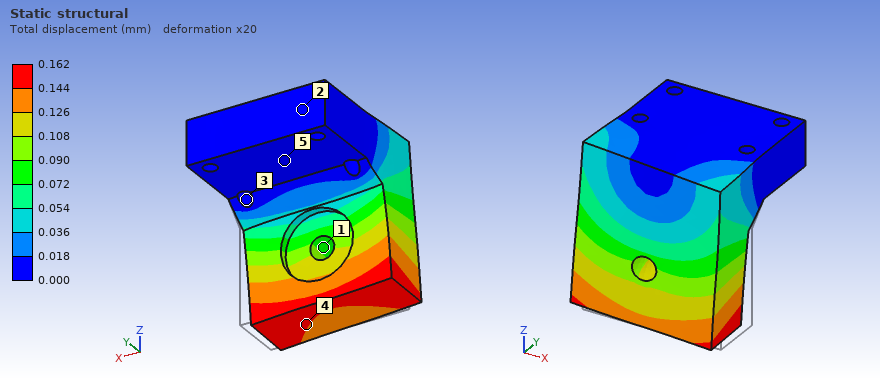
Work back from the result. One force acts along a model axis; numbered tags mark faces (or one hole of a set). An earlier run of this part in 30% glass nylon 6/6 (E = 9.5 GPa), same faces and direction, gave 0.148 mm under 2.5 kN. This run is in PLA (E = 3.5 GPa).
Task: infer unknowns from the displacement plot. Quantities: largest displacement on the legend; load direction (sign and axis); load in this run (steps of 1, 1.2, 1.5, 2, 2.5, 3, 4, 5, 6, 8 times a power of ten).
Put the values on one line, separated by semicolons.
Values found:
0.162 mm; -X; 1 kN
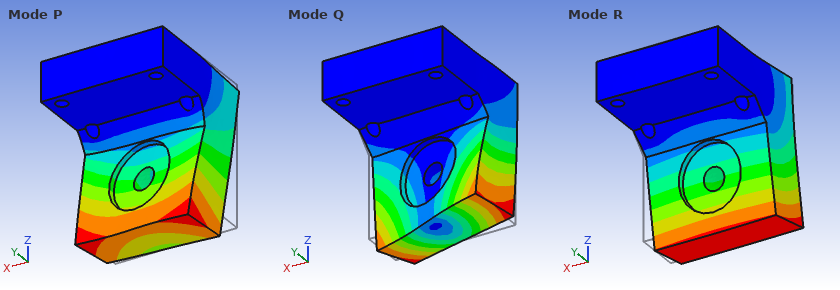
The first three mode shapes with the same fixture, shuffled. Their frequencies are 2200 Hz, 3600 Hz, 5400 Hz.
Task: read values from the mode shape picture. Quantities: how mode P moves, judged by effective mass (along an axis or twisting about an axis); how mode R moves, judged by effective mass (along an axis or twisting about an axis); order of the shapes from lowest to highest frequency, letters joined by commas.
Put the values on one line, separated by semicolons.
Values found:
along X; along Y; R, P, Q
